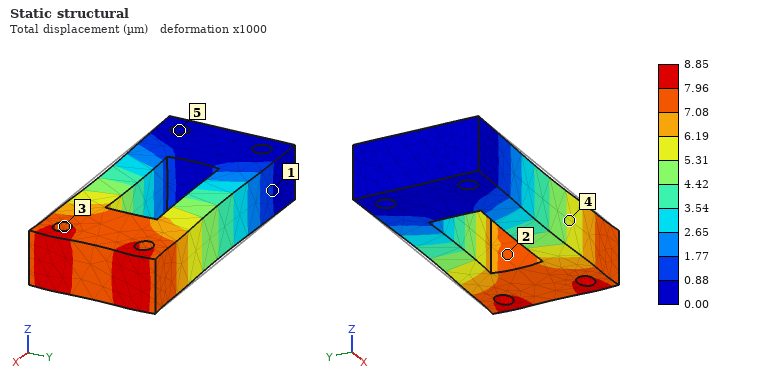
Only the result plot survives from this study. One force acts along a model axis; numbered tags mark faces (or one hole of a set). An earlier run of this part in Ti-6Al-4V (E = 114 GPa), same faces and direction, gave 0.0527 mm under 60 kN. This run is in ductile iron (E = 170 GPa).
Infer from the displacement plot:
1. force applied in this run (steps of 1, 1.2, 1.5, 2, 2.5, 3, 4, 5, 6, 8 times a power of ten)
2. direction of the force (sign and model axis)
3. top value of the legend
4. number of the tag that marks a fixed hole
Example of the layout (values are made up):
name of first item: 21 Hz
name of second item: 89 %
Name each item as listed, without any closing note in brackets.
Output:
force applied in this run: 15 kN
direction of the force: +X
top value of the legend: 8.85 µm
number of the tag that marks a fixed hole: 5
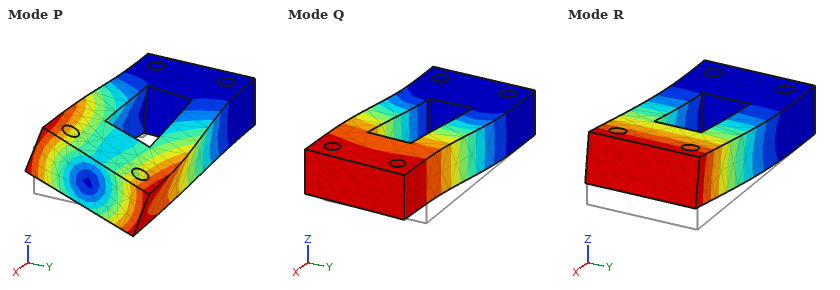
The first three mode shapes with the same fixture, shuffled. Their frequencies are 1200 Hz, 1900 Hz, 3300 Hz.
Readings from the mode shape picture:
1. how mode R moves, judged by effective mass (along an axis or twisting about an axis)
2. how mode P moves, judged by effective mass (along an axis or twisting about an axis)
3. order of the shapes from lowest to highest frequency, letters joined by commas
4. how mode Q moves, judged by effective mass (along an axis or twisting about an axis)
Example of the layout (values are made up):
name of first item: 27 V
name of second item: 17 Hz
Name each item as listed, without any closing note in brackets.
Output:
how mode R moves, judged by effective mass: along Z
how mode P moves, judged by effective mass: twisting about X
order of the shapes from lowest to highest frequency, letters joined by commas: R, Q, P
how mode Q moves, judged by effective mass: along Y
